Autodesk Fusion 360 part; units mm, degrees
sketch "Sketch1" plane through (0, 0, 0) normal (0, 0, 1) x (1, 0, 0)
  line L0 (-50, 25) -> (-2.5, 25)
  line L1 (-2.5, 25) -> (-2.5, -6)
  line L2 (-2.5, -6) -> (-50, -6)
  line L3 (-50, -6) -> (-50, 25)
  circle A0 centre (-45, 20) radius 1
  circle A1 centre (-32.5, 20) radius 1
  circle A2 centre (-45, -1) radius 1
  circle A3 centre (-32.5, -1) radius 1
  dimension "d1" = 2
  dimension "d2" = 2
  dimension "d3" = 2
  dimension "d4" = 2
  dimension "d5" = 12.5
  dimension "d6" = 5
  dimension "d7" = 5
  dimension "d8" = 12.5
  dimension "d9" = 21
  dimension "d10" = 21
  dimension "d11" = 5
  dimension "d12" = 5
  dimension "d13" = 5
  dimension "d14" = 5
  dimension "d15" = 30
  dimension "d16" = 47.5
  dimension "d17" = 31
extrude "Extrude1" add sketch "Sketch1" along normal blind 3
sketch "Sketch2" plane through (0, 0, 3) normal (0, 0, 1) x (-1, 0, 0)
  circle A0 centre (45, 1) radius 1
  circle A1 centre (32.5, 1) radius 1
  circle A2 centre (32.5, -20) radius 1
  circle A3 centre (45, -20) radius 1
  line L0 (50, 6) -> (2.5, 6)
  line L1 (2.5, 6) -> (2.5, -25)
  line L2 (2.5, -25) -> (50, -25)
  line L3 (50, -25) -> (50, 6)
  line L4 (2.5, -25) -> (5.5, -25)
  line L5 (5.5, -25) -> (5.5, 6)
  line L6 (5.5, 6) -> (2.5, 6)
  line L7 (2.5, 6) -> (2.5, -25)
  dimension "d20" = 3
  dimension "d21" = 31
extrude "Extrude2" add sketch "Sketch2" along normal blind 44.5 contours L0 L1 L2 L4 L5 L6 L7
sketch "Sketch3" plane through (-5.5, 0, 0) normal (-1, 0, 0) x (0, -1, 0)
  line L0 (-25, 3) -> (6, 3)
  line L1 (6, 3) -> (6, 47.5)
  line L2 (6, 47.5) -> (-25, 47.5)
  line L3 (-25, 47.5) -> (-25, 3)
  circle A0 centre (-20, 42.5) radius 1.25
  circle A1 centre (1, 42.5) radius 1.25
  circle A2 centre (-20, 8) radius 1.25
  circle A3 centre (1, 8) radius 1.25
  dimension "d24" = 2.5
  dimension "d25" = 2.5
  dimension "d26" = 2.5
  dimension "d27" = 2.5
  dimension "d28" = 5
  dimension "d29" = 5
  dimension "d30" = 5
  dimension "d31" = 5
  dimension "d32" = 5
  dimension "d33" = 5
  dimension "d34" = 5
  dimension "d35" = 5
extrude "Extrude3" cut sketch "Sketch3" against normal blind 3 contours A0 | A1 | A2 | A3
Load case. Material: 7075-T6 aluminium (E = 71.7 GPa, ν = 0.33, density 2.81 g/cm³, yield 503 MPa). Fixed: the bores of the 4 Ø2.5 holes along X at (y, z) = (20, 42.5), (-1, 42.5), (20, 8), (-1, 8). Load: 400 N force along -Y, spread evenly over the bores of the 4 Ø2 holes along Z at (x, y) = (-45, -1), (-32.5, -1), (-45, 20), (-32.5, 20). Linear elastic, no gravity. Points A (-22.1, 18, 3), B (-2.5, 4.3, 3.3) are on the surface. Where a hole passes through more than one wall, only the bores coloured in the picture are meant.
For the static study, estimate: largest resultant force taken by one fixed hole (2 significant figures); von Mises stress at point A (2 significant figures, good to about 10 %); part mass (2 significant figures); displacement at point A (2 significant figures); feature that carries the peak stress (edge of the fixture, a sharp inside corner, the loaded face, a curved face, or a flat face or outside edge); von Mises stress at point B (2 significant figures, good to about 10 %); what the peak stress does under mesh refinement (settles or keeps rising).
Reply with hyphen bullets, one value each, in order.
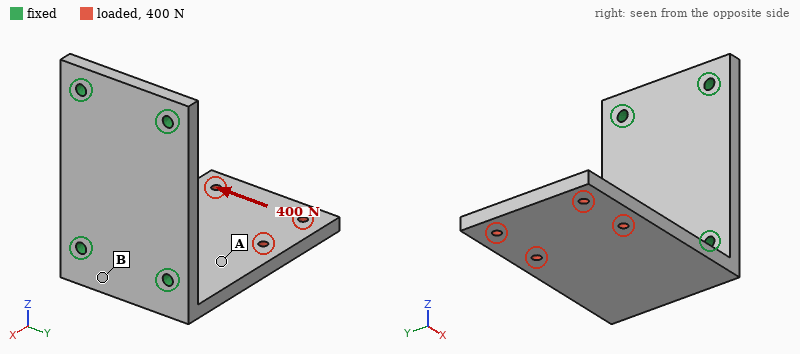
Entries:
- 670 N
- 17 MPa
- 24 g
- 0.053 mm
- edge of the fixture
- 44 MPa
- keeps rising
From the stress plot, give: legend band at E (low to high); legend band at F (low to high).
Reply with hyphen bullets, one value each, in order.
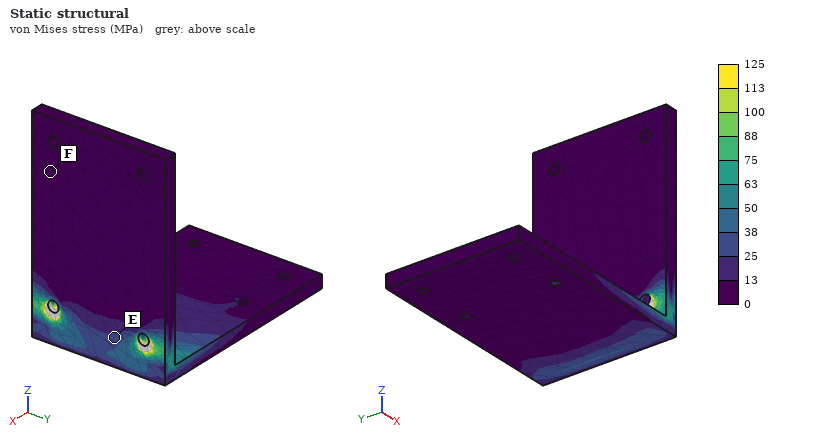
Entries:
- 25 to 38 MPa
- 0 to 13 MPa
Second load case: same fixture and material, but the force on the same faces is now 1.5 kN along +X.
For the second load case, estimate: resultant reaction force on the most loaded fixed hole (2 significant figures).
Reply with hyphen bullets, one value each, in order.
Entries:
- 780 N
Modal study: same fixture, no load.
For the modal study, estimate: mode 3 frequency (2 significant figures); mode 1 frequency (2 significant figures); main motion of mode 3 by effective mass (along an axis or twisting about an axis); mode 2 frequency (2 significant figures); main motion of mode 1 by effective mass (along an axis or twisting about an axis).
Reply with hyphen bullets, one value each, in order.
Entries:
- 4400 Hz
- 970 Hz
- along Y
- 3300 Hz
- along Z
